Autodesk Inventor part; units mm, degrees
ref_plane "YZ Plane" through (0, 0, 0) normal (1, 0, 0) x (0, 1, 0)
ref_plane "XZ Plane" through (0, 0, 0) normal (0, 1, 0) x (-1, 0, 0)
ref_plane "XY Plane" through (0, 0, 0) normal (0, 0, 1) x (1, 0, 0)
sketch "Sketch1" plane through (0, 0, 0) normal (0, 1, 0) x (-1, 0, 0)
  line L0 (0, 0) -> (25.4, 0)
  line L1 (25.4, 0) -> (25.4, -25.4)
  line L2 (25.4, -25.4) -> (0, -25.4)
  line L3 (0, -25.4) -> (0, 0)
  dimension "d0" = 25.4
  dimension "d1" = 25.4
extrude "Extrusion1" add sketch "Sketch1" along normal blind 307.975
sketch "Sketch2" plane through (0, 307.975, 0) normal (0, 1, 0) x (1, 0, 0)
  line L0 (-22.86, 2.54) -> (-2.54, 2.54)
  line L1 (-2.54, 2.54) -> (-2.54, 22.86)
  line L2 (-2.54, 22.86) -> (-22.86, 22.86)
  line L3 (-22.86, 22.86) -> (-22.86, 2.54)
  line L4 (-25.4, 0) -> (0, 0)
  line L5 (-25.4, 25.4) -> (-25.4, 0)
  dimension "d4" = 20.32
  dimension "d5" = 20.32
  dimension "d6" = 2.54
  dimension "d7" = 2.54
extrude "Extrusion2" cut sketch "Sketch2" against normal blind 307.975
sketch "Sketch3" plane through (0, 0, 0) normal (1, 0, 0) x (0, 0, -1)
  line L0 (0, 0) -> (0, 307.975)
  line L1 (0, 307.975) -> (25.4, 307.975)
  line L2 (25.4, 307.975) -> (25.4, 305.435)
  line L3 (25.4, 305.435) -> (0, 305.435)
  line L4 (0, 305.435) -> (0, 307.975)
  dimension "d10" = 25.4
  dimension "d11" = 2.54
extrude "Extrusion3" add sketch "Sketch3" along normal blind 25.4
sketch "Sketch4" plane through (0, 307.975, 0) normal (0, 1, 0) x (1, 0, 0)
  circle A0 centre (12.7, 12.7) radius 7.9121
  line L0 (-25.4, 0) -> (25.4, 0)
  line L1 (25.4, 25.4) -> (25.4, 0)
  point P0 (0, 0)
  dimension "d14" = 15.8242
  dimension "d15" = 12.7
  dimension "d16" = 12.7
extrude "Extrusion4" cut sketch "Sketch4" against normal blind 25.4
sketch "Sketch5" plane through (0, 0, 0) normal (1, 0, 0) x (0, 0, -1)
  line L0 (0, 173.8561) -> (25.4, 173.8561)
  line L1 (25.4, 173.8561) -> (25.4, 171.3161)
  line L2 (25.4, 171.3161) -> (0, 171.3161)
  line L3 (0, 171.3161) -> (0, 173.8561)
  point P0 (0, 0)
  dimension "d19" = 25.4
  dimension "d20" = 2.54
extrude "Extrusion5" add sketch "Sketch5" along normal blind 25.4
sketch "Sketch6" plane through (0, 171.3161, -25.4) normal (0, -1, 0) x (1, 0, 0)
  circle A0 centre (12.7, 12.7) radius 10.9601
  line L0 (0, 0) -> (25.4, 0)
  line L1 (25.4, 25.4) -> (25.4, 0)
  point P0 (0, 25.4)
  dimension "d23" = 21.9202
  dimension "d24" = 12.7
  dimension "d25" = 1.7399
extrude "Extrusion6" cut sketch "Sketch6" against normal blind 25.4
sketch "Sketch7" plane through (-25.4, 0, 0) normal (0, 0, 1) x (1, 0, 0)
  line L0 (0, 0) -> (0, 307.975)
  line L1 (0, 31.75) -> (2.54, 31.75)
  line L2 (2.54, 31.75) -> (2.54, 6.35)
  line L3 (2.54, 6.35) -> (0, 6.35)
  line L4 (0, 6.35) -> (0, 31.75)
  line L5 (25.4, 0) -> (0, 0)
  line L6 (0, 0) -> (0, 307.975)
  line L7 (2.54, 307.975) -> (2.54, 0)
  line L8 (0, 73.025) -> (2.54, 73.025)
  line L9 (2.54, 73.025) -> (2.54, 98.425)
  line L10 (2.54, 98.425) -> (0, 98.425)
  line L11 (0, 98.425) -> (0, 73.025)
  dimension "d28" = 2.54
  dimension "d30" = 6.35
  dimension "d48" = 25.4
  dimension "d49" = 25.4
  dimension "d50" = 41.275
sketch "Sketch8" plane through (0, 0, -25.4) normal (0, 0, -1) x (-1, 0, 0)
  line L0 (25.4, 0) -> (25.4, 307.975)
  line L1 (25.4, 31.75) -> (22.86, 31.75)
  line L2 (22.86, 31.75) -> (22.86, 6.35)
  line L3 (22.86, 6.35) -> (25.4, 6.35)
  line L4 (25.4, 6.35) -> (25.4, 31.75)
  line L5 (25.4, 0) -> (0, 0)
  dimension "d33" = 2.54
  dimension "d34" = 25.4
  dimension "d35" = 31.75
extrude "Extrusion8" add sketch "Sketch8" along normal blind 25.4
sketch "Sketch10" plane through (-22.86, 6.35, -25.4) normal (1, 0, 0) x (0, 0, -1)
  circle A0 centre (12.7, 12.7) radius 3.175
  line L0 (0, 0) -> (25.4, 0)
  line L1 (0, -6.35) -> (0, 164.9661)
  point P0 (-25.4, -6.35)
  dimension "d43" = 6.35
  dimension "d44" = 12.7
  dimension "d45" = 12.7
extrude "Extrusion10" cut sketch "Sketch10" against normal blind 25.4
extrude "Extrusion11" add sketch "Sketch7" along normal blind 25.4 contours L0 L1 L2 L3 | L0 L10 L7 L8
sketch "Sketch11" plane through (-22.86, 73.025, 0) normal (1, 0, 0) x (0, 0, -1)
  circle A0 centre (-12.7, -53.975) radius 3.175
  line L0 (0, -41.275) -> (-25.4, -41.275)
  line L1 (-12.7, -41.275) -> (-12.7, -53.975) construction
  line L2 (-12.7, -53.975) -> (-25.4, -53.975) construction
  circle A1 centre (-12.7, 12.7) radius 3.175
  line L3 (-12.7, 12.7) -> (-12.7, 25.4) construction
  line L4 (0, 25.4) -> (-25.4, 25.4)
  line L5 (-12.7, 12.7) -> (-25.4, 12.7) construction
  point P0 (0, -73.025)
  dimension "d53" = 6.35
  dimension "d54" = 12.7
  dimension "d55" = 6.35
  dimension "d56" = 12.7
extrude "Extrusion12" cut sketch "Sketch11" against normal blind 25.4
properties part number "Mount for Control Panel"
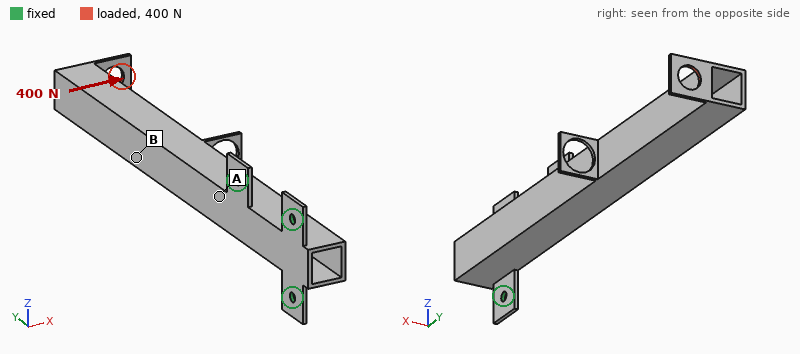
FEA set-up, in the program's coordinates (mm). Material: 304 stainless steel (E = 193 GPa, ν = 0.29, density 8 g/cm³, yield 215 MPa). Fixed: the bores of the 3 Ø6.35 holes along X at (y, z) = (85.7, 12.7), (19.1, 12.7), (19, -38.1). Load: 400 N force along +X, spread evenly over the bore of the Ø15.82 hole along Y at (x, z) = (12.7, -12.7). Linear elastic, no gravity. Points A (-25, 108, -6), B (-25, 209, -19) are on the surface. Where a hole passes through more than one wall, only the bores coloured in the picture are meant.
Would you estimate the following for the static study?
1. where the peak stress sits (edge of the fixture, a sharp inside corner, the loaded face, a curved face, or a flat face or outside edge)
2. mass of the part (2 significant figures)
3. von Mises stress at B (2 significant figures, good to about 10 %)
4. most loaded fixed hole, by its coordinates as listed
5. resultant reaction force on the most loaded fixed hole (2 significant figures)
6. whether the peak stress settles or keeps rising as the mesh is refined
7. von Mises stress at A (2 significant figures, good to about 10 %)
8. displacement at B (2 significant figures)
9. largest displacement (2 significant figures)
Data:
edge of the fixture
620 g
25 MPa
(85.7, 12.7)
1.7 kN
keeps rising
58 MPa
0.58 mm
1.1 mm
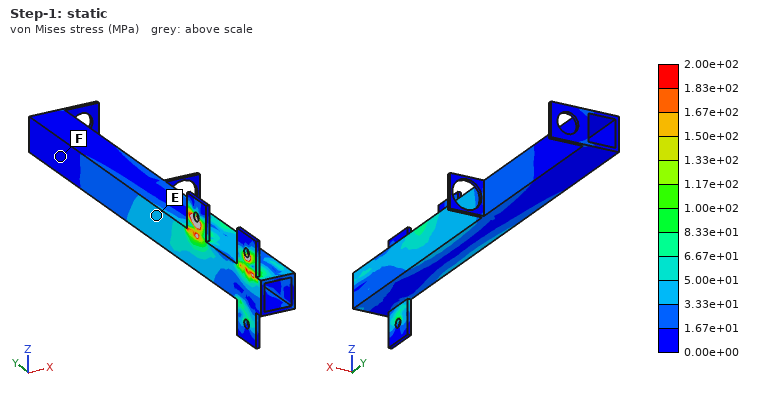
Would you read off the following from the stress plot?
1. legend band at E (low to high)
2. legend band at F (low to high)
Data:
3.33e+01 to 5.00e+01 MPa
0.00e+00 to 1.67e+01 MPa
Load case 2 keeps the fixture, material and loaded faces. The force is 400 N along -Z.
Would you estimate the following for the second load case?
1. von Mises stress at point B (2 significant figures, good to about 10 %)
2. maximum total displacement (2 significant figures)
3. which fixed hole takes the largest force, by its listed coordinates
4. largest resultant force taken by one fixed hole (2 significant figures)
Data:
12 MPa
0.65 mm
(85.7, 12.7)
1.6 kN
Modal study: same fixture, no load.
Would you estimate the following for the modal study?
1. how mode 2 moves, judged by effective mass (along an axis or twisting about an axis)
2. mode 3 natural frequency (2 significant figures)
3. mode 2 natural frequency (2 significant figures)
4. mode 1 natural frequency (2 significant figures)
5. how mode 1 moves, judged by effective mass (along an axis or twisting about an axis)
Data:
along Z
1300 Hz
400 Hz
250 Hz
along X
